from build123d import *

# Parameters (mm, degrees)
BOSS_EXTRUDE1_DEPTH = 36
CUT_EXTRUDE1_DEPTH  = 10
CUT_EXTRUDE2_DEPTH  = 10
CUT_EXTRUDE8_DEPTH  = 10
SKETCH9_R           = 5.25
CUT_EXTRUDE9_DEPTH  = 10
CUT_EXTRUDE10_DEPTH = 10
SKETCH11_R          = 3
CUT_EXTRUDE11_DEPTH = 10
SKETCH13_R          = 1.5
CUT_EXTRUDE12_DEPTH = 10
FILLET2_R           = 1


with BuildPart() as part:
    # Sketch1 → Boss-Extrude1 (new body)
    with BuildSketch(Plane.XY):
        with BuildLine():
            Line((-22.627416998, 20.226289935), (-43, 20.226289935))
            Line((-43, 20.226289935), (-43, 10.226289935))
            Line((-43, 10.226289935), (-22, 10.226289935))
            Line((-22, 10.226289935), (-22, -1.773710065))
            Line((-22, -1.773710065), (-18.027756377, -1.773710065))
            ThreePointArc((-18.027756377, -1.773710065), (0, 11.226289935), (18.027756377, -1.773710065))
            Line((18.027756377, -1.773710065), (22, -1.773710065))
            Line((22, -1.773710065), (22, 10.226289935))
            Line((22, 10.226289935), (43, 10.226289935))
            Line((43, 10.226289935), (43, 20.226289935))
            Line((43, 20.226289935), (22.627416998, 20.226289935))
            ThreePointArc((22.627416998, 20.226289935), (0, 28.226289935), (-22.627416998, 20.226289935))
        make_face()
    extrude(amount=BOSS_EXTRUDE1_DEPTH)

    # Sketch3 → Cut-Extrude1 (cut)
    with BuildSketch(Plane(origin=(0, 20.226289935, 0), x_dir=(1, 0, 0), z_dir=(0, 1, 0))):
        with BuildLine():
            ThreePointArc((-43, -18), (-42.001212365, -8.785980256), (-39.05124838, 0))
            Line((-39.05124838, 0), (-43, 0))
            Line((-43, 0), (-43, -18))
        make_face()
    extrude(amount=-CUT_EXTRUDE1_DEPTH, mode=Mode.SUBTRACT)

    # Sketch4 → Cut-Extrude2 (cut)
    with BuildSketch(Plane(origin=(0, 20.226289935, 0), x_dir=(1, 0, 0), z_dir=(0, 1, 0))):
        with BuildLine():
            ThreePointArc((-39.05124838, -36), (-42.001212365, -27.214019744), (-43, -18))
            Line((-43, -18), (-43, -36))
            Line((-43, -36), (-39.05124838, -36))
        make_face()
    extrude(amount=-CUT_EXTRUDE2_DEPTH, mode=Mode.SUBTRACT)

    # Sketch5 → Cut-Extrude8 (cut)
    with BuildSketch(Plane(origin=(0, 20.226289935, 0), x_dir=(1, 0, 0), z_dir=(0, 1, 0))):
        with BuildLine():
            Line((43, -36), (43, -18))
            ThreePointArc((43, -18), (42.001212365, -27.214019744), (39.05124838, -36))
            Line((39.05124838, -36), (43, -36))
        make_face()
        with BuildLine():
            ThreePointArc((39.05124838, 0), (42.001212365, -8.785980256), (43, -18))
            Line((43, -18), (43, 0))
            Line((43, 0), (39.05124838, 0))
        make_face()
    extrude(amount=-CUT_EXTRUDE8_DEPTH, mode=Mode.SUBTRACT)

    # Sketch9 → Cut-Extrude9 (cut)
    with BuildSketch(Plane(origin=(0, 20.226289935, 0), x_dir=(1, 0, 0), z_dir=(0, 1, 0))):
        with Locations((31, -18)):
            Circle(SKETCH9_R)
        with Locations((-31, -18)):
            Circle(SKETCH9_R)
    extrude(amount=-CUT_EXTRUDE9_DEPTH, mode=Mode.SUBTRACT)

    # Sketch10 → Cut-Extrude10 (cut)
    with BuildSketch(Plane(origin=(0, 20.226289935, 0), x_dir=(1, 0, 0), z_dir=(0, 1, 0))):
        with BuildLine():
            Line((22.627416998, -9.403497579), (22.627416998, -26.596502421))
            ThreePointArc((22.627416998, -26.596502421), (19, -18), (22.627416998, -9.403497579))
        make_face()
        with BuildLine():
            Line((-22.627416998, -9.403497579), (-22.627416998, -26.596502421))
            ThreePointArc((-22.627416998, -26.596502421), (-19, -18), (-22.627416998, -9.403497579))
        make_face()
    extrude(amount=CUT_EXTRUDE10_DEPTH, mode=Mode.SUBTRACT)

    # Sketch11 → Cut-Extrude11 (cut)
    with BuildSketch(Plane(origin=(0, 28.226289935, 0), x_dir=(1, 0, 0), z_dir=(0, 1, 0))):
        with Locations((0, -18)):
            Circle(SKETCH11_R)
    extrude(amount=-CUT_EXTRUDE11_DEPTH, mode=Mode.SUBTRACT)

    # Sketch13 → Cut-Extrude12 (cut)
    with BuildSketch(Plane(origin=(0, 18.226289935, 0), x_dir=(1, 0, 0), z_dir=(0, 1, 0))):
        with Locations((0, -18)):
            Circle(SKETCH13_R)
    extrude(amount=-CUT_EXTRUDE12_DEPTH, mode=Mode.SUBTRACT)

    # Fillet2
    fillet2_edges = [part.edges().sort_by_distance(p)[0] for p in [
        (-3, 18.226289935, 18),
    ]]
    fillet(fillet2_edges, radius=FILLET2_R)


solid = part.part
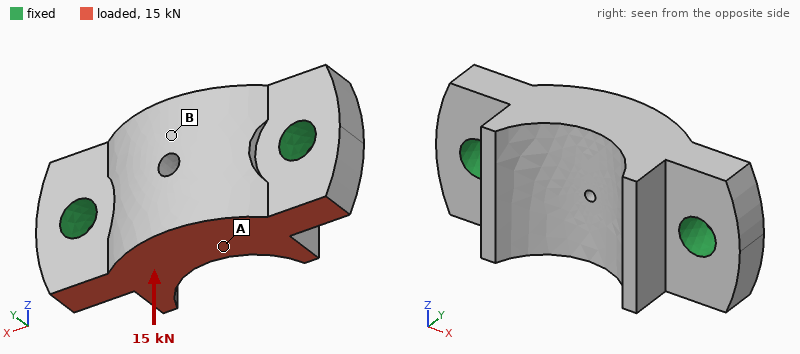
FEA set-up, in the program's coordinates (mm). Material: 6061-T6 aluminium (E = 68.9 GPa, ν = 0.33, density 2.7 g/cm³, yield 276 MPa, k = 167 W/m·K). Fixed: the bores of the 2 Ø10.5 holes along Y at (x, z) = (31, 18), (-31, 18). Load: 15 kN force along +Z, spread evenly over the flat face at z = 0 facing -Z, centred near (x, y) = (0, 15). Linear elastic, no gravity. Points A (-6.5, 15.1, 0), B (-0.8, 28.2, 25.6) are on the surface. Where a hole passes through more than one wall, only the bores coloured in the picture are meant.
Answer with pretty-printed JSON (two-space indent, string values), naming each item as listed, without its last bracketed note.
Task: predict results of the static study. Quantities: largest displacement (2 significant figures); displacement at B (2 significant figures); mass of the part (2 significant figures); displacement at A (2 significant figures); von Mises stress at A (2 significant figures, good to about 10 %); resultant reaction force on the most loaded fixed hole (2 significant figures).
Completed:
{
  "largest displacement": "22 µm",
  "displacement at B": "17 µm",
  "mass of the part": "120 g",
  "displacement at A": "16 µm",
  "von Mises stress at A": "24 MPa",
  "resultant reaction force on the most loaded fixed hole": "7.5 kN"
}
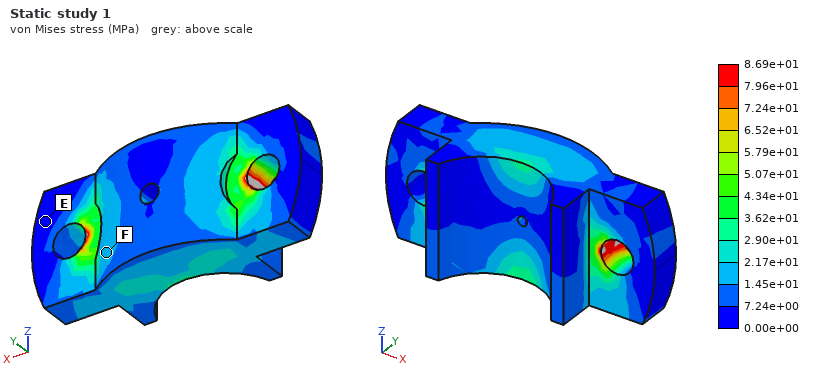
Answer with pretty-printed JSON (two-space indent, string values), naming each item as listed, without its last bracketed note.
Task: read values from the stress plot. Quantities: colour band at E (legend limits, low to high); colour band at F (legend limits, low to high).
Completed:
{
  "colour band at E": "0.00e+00 to 7.24e+00 MPa",
  "colour band at F": "1.45e+01 to 2.17e+01 MPa"
}
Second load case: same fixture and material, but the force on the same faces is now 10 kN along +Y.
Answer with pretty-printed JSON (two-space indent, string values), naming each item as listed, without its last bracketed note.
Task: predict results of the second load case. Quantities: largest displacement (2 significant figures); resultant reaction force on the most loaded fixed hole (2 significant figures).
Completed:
{
  "largest displacement": "79 µm",
  "resultant reaction force on the most loaded fixed hole": "5.1 kN"
}
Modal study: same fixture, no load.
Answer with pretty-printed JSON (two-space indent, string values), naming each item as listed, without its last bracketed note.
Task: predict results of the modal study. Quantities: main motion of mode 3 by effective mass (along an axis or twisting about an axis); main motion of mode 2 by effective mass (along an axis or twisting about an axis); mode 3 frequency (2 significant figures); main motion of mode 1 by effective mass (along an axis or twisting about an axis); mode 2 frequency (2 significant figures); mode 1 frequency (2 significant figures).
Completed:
{
  "main motion of mode 3 by effective mass": "along Z",
  "main motion of mode 2 by effective mass": "along Y",
  "mode 3 frequency": "16 kHz",
  "main motion of mode 1 by effective mass": "twisting about X",
  "mode 2 frequency": "12 kHz",
  "mode 1 frequency": "11 kHz"
}
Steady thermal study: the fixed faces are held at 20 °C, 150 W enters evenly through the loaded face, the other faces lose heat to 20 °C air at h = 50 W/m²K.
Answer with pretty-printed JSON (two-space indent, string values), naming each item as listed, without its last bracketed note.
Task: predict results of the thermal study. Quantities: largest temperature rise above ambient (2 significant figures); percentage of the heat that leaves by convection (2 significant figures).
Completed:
{
  "largest temperature rise above ambient": "24 K",
  "percentage of the heat that leaves by convection": "3.0 %"
}
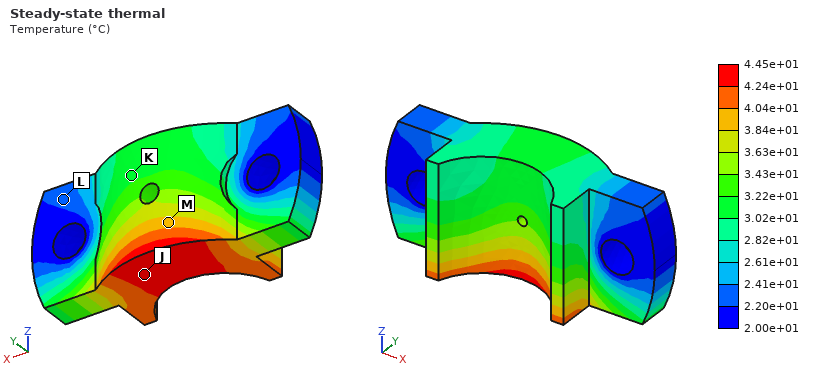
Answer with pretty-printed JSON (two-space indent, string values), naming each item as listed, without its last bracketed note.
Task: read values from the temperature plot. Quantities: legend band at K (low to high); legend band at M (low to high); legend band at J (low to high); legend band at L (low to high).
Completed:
{
  "legend band at K": "3.02e+01 to 3.22e+01 °C",
  "legend band at M": "3.84e+01 to 4.04e+01 °C",
  "legend band at J": "4.24e+01 to 4.45e+01 °C",
  "legend band at L": "2.20e+01 to 2.41e+01 °C"
}
